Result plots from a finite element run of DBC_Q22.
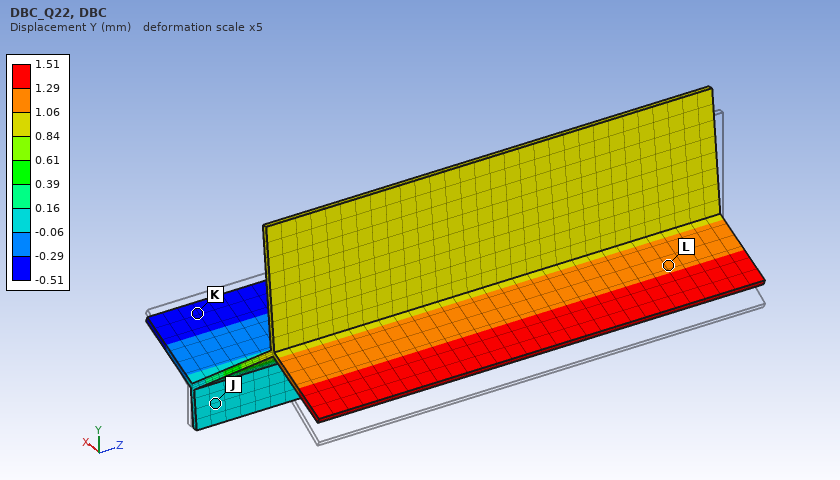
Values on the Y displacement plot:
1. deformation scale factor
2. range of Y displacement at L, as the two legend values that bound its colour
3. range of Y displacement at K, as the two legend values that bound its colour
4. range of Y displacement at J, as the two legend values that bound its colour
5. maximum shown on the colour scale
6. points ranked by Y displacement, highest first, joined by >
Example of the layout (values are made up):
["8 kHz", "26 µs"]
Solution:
["5", "1.06 to 1.29 mm", "-0.51 to -0.29 mm", "-0.06 to 0.16 mm", "1.51 mm", "L > J > K"]
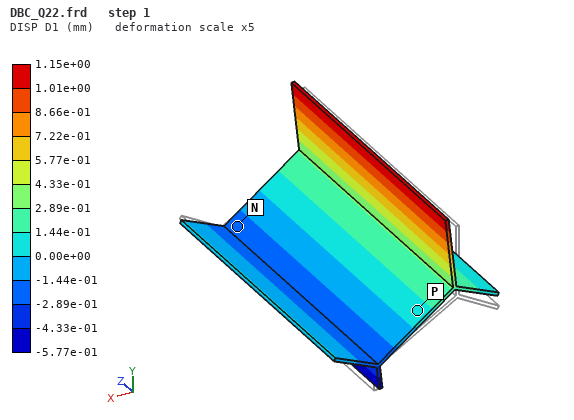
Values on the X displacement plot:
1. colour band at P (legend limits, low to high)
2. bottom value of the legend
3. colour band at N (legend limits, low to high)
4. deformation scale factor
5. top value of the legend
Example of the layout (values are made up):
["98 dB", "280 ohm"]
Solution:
["0.00e+00 to 1.44e-01 mm", "-5.77e-01 mm", "-2.89e-01 to -1.44e-01 mm", "5", "1.15e+00 mm"]
